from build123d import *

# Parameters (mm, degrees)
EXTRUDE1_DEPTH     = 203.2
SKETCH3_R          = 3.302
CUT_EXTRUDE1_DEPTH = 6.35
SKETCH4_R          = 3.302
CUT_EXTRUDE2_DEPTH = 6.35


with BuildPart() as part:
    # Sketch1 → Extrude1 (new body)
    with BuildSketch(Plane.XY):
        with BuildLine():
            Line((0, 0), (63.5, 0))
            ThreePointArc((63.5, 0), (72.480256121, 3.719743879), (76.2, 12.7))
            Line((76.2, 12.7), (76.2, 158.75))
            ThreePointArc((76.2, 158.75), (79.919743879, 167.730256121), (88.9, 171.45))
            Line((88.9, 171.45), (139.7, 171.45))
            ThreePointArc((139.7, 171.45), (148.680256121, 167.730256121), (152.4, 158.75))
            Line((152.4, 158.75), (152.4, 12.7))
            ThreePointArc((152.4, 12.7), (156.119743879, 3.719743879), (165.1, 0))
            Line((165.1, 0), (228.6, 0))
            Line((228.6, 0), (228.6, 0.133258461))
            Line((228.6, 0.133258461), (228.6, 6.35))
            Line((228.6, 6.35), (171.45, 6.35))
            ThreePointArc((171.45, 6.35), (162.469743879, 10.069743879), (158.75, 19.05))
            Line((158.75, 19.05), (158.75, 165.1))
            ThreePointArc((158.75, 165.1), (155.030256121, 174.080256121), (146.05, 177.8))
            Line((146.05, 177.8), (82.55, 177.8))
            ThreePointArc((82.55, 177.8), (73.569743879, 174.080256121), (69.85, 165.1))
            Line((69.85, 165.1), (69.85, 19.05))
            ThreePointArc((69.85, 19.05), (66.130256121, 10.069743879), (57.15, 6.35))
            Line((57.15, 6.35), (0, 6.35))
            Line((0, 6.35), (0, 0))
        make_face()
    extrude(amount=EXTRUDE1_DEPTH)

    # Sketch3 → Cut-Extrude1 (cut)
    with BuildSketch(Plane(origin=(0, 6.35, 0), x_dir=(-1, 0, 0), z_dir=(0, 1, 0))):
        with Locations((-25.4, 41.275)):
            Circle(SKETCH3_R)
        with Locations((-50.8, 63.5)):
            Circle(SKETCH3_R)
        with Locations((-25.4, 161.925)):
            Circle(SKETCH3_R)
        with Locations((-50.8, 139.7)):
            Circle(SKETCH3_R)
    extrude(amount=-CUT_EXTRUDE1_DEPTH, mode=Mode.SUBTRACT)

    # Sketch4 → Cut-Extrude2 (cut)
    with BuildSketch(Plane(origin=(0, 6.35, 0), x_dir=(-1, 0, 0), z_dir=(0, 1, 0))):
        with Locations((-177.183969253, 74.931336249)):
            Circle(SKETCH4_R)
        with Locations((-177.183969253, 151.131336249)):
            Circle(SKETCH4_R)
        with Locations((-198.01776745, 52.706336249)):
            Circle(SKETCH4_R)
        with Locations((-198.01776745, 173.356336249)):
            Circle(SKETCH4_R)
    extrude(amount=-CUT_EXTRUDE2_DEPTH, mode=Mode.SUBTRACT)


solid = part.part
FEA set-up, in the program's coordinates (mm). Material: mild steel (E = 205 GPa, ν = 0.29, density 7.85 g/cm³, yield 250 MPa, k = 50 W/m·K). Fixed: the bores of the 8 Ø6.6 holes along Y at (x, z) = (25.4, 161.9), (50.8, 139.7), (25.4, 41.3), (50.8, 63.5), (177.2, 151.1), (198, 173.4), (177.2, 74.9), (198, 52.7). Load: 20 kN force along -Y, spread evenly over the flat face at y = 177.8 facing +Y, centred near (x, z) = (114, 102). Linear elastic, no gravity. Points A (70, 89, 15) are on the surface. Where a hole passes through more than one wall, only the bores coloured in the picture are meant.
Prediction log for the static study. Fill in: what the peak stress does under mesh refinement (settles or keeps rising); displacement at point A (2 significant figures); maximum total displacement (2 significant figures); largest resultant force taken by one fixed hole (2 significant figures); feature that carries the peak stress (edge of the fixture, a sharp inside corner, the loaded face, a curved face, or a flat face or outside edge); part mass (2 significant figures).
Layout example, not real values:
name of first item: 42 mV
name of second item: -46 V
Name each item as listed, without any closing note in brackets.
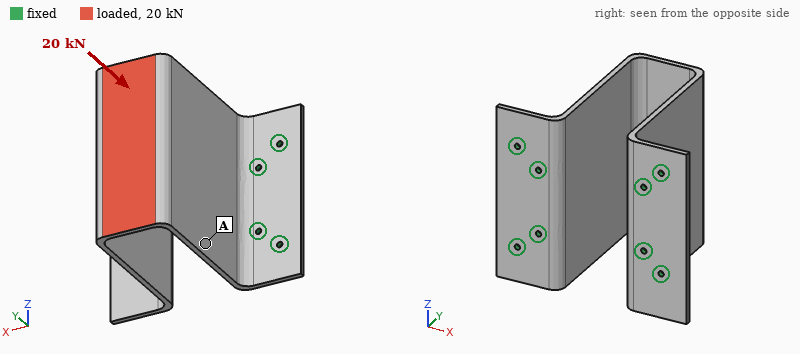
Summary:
what the peak stress does under mesh refinement: keeps rising
displacement at point A: 0.076 mm
maximum total displacement: 0.17 mm
largest resultant force taken by one fixed hole: 6.1 kN
feature that carries the peak stress: edge of the fixture
part mass: 5.8 kg
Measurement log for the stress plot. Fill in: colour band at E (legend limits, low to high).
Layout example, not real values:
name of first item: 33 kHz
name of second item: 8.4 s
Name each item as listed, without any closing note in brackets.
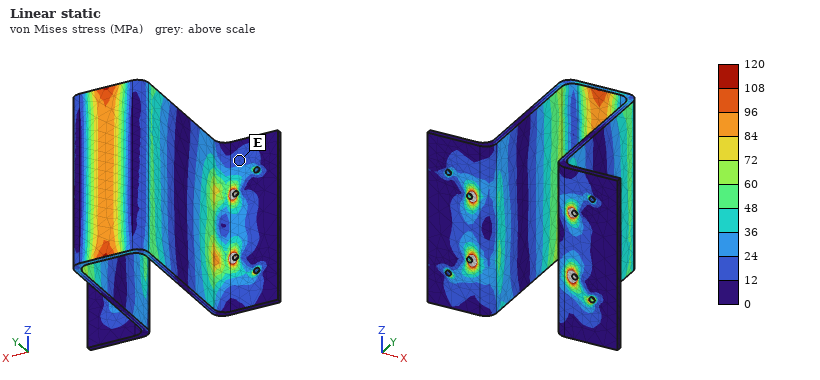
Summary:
colour band at E: 12 to 24 MPa
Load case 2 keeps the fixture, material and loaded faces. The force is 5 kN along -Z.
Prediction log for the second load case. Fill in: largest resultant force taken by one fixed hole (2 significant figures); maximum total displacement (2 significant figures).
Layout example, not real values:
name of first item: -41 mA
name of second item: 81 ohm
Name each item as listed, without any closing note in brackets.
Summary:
largest resultant force taken by one fixed hole: 5.1 kN
maximum total displacement: 0.22 mm
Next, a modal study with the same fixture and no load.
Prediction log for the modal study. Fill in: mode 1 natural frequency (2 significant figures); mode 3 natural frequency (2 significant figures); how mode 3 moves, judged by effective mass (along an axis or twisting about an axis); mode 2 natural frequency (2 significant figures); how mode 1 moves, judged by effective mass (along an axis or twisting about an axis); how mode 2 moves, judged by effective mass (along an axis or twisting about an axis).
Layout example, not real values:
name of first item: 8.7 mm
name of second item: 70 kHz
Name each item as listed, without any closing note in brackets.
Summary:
mode 1 natural frequency: 220 Hz
mode 3 natural frequency: 520 Hz
how mode 3 moves, judged by effective mass: along Z
mode 2 natural frequency: 400 Hz
how mode 1 moves, judged by effective mass: along X
how mode 2 moves, judged by effective mass: twisting about Y
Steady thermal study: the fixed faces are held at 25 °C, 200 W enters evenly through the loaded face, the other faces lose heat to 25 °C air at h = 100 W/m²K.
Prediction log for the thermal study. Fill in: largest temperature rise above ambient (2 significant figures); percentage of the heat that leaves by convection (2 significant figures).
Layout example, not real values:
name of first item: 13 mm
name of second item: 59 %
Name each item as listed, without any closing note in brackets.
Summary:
largest temperature rise above ambient: 55 K
percentage of the heat that leaves by convection: 99 %
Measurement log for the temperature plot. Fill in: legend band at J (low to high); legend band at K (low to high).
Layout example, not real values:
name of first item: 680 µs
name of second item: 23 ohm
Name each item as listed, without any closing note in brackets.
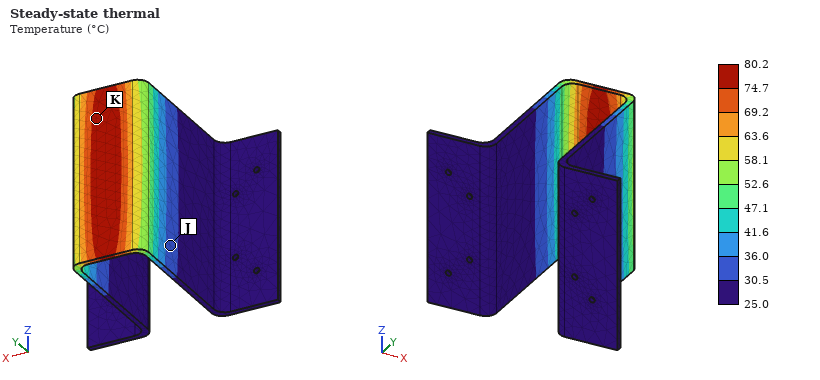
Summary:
legend band at J: 30.5 to 36.0 °C
legend band at K: 74.7 to 80.2 °C
